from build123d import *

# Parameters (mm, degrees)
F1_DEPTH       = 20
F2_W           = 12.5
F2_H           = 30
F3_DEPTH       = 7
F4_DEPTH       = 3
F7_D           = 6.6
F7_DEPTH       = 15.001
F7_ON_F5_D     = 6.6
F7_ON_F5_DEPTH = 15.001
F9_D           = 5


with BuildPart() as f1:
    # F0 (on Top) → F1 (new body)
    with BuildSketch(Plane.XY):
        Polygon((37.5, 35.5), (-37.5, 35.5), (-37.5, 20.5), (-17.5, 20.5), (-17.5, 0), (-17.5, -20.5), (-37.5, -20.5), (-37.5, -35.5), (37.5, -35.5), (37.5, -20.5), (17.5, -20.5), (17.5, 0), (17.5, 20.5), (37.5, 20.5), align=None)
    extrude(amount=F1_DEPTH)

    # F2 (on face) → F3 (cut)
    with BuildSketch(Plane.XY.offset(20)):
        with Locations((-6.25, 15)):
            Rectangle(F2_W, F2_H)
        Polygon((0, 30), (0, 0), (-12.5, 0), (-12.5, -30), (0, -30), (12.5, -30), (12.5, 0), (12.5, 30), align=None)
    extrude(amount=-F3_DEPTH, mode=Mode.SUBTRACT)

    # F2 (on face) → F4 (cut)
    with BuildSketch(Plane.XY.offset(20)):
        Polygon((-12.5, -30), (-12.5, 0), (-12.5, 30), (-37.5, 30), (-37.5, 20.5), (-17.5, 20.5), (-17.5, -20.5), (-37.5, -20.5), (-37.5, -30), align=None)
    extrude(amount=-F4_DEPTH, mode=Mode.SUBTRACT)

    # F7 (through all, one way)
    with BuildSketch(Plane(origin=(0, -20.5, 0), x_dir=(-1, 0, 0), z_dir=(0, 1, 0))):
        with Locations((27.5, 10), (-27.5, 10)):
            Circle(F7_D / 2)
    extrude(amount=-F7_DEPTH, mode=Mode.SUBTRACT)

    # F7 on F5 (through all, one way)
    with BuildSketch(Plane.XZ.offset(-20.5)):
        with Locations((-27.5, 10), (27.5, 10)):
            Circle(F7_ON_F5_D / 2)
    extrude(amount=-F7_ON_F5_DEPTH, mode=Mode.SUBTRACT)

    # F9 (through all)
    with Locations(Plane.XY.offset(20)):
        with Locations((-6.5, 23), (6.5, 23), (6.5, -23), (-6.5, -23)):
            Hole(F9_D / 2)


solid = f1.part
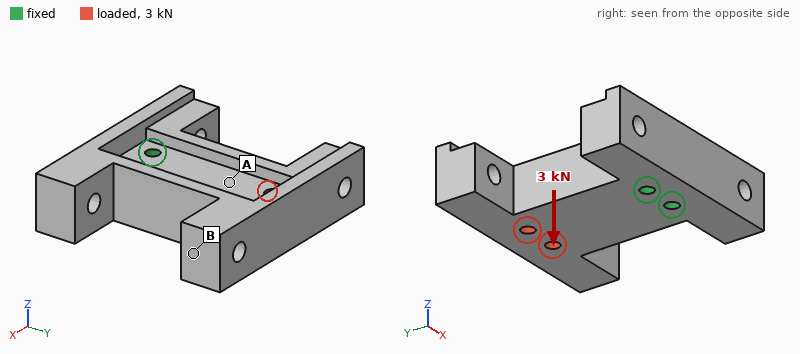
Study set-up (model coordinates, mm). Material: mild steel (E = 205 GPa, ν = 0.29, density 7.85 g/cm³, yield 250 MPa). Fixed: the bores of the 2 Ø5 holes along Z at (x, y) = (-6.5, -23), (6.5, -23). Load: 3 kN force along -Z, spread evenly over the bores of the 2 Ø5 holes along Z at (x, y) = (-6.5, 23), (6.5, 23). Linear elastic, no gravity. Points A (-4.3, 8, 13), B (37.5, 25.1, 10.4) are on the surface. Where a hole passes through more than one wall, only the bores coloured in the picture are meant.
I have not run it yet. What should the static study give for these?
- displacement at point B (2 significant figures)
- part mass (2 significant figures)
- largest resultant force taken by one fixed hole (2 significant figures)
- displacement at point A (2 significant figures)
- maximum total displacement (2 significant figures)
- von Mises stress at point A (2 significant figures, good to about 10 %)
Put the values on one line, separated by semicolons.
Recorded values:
58 µm; 460 g; 1.5 kN; 34 µm; 82 µm; 24 MPa
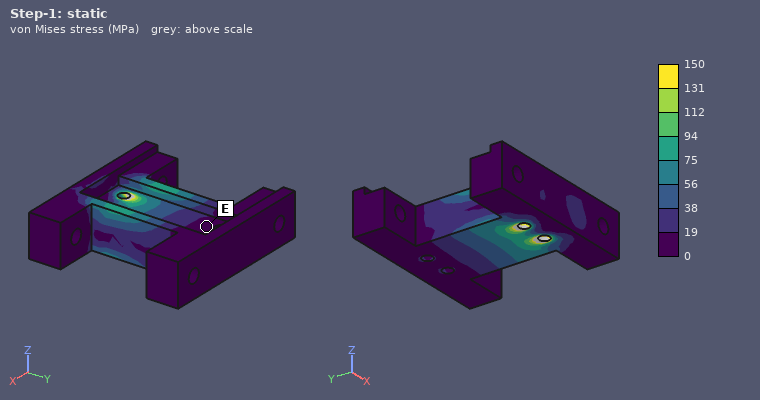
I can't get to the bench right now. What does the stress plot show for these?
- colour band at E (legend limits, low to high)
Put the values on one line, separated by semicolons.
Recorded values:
0 to 19 MPa
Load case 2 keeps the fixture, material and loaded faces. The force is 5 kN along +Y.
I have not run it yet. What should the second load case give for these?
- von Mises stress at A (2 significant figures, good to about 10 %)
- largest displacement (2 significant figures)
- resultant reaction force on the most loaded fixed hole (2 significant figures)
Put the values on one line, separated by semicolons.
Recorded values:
10 MPa; 4.1 µm; 2.5 kN
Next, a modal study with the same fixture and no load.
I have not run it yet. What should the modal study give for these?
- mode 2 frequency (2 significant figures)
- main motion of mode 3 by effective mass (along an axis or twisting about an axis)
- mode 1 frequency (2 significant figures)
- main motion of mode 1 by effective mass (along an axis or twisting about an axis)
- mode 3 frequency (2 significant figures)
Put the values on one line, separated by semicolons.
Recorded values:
3200 Hz; along X; 2300 Hz; along Z; 3800 Hz
